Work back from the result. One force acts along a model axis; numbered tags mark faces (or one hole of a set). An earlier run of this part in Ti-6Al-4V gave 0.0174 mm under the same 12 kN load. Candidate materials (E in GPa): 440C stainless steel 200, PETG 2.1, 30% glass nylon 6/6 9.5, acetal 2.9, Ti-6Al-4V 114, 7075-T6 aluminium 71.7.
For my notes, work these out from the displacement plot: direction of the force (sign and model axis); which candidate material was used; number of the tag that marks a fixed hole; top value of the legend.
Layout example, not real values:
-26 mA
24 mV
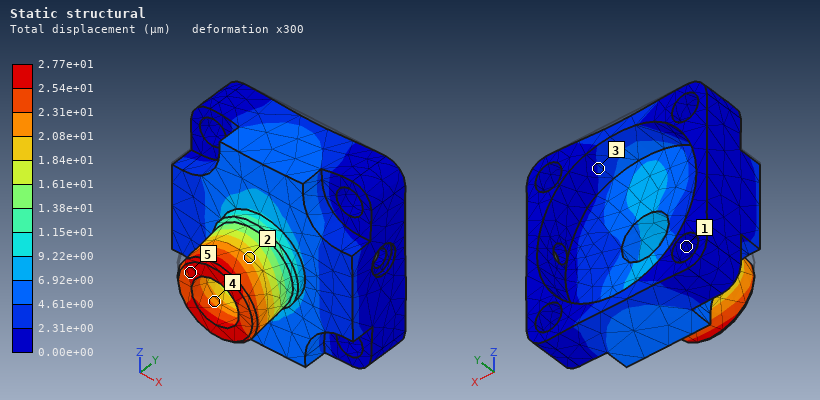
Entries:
-Z
7075-T6 aluminium
1
2.77e+01 µm
